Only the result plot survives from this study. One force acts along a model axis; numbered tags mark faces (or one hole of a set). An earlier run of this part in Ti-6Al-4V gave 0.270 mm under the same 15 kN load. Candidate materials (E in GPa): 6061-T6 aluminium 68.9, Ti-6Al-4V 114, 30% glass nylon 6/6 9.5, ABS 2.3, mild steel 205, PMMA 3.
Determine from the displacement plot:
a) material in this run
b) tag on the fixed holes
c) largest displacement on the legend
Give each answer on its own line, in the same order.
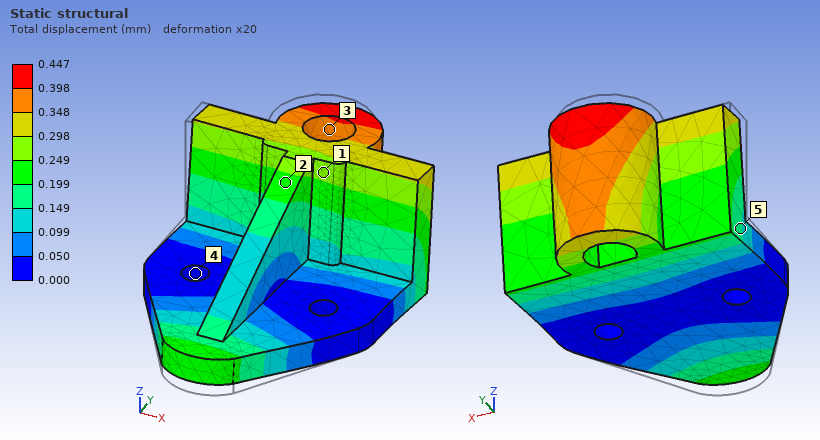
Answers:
6061-T6 aluminium
4
0.447 mm
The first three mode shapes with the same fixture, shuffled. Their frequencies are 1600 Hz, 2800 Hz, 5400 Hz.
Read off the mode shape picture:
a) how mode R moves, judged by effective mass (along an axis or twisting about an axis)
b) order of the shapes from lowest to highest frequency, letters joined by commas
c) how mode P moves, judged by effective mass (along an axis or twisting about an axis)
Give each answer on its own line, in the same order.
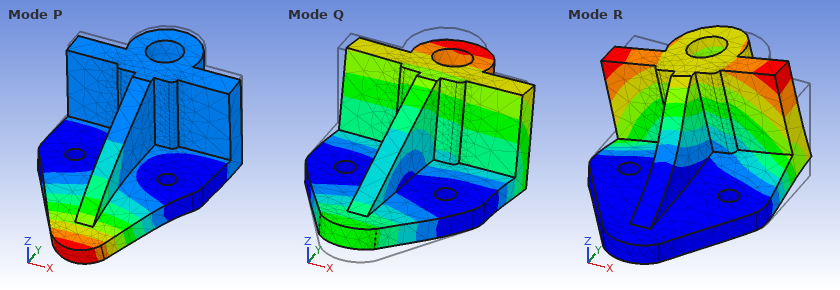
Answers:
along X
Q, R, P
along Z
